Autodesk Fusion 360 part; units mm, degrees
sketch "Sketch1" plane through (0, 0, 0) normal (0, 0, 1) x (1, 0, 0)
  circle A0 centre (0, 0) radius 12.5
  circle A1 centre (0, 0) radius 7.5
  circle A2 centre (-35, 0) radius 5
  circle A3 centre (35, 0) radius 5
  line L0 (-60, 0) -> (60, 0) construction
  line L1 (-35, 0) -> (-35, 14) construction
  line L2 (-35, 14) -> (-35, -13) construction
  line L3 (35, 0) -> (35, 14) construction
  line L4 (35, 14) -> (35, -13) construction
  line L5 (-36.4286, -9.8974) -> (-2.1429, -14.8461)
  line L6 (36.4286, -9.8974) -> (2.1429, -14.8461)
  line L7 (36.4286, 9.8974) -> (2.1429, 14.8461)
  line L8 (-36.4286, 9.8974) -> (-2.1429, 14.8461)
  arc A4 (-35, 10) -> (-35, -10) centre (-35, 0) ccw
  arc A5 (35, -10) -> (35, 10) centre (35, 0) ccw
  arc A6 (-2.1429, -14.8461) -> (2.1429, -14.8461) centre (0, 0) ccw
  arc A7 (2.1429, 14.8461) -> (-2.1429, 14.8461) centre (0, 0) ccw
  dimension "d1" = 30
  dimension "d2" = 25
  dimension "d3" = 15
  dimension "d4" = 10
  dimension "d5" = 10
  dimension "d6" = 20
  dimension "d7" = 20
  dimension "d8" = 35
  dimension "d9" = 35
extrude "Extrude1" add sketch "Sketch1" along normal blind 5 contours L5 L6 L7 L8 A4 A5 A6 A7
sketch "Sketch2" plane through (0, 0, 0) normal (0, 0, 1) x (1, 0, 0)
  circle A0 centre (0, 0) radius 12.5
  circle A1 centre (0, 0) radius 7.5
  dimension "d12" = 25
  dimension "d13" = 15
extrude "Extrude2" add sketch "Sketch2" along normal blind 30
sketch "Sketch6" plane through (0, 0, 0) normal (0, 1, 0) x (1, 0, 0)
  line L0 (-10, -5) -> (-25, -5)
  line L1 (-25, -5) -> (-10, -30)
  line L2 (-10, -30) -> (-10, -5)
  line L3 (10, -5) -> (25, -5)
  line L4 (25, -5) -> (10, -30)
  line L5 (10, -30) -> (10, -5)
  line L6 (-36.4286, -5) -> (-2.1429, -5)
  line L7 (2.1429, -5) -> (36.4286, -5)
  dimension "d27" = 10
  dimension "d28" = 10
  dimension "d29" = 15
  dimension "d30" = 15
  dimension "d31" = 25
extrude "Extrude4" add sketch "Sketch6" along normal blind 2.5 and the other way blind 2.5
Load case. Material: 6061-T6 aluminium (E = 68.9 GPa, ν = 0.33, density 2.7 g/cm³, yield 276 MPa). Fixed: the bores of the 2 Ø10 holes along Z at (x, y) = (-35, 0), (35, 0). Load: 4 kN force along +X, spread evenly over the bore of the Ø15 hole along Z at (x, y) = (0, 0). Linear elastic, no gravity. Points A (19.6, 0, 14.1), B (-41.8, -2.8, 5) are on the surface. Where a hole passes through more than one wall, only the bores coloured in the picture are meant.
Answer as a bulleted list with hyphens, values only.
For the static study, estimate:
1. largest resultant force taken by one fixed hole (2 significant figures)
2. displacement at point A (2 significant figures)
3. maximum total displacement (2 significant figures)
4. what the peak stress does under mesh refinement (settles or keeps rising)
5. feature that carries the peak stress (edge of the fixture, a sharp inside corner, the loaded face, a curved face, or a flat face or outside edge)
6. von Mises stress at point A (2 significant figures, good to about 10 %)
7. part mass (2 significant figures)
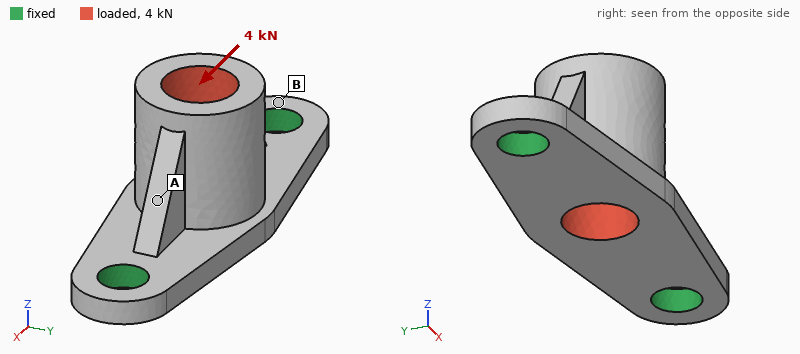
- 2.2 kN
- 16 µm
- 28 µm
- keeps rising
- edge of the fixture
- 31 MPa
- 48 g
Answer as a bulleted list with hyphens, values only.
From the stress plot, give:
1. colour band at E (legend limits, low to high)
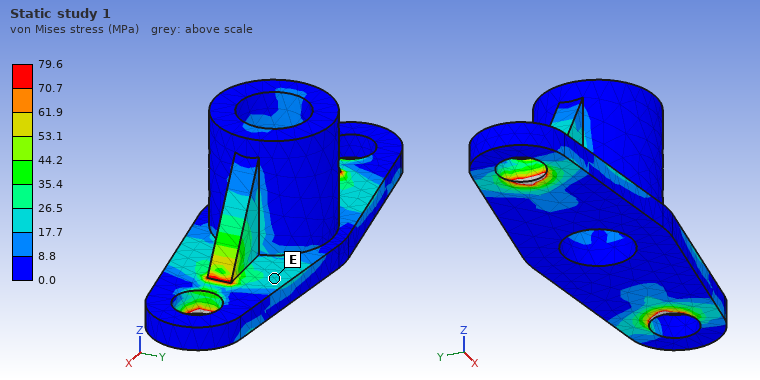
- 17.7 to 26.5 MPa
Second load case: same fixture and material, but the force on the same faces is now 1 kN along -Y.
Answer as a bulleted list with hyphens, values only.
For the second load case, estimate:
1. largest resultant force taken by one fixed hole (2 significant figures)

- 500 N
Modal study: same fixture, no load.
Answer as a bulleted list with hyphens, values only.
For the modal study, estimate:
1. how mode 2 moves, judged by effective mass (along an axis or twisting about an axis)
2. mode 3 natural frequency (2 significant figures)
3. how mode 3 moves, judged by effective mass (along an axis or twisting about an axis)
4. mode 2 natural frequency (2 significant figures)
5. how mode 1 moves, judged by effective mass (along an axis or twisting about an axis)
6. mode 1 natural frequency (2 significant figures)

- along Z
- 12 kHz
- along X
- 7200 Hz
- along Y
- 3100 Hz
